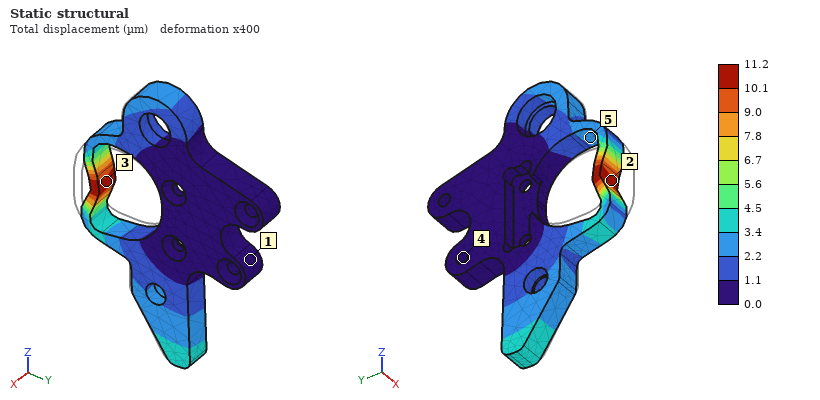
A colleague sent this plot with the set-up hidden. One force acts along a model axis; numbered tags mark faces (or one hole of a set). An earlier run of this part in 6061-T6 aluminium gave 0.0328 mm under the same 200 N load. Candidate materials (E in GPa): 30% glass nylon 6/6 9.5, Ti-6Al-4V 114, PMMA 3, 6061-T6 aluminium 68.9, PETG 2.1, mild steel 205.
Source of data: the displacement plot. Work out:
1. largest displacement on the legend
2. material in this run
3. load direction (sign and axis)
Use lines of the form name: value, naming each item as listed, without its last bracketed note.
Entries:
largest displacement on the legend: 11.2 µm
material in this run: mild steel
load direction: +Y
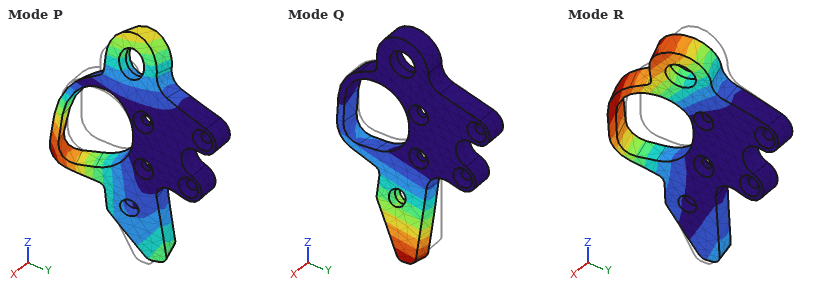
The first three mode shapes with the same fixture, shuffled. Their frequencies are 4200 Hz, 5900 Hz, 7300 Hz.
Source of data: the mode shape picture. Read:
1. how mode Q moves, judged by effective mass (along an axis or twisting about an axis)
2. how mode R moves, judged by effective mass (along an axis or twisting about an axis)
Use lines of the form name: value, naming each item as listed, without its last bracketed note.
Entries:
how mode Q moves, judged by effective mass: along X
how mode R moves, judged by effective mass: along X
